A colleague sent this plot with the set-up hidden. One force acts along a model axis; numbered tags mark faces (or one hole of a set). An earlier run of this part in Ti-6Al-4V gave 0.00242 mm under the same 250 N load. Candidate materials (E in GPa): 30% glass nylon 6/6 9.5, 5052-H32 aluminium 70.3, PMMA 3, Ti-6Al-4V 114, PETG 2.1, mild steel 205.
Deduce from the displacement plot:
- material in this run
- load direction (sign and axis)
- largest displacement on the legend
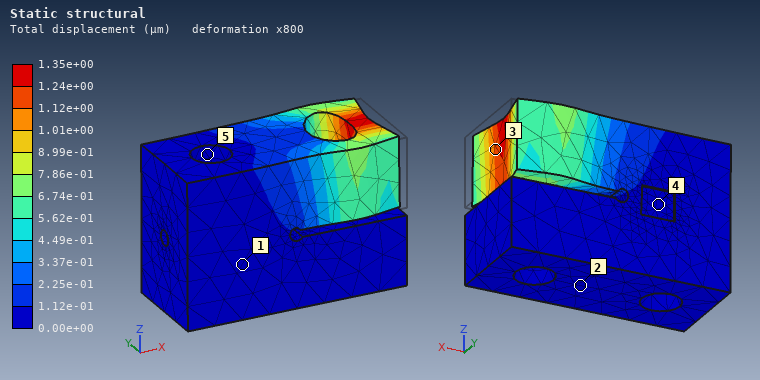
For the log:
mild steel
-X
1.35e+00 µm
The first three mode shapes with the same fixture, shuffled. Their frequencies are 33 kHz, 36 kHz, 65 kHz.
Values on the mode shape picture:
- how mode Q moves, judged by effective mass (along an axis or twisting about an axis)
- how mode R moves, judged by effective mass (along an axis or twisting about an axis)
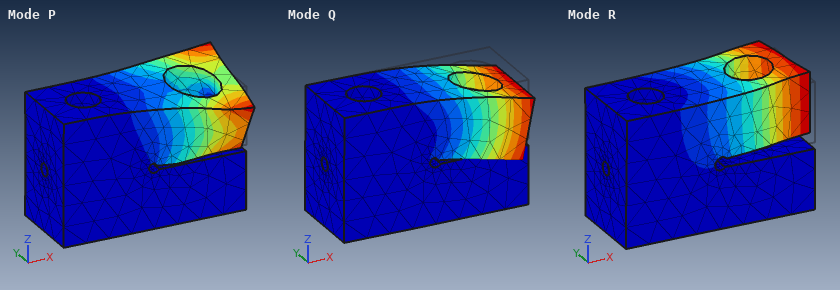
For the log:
along Z
along Y
